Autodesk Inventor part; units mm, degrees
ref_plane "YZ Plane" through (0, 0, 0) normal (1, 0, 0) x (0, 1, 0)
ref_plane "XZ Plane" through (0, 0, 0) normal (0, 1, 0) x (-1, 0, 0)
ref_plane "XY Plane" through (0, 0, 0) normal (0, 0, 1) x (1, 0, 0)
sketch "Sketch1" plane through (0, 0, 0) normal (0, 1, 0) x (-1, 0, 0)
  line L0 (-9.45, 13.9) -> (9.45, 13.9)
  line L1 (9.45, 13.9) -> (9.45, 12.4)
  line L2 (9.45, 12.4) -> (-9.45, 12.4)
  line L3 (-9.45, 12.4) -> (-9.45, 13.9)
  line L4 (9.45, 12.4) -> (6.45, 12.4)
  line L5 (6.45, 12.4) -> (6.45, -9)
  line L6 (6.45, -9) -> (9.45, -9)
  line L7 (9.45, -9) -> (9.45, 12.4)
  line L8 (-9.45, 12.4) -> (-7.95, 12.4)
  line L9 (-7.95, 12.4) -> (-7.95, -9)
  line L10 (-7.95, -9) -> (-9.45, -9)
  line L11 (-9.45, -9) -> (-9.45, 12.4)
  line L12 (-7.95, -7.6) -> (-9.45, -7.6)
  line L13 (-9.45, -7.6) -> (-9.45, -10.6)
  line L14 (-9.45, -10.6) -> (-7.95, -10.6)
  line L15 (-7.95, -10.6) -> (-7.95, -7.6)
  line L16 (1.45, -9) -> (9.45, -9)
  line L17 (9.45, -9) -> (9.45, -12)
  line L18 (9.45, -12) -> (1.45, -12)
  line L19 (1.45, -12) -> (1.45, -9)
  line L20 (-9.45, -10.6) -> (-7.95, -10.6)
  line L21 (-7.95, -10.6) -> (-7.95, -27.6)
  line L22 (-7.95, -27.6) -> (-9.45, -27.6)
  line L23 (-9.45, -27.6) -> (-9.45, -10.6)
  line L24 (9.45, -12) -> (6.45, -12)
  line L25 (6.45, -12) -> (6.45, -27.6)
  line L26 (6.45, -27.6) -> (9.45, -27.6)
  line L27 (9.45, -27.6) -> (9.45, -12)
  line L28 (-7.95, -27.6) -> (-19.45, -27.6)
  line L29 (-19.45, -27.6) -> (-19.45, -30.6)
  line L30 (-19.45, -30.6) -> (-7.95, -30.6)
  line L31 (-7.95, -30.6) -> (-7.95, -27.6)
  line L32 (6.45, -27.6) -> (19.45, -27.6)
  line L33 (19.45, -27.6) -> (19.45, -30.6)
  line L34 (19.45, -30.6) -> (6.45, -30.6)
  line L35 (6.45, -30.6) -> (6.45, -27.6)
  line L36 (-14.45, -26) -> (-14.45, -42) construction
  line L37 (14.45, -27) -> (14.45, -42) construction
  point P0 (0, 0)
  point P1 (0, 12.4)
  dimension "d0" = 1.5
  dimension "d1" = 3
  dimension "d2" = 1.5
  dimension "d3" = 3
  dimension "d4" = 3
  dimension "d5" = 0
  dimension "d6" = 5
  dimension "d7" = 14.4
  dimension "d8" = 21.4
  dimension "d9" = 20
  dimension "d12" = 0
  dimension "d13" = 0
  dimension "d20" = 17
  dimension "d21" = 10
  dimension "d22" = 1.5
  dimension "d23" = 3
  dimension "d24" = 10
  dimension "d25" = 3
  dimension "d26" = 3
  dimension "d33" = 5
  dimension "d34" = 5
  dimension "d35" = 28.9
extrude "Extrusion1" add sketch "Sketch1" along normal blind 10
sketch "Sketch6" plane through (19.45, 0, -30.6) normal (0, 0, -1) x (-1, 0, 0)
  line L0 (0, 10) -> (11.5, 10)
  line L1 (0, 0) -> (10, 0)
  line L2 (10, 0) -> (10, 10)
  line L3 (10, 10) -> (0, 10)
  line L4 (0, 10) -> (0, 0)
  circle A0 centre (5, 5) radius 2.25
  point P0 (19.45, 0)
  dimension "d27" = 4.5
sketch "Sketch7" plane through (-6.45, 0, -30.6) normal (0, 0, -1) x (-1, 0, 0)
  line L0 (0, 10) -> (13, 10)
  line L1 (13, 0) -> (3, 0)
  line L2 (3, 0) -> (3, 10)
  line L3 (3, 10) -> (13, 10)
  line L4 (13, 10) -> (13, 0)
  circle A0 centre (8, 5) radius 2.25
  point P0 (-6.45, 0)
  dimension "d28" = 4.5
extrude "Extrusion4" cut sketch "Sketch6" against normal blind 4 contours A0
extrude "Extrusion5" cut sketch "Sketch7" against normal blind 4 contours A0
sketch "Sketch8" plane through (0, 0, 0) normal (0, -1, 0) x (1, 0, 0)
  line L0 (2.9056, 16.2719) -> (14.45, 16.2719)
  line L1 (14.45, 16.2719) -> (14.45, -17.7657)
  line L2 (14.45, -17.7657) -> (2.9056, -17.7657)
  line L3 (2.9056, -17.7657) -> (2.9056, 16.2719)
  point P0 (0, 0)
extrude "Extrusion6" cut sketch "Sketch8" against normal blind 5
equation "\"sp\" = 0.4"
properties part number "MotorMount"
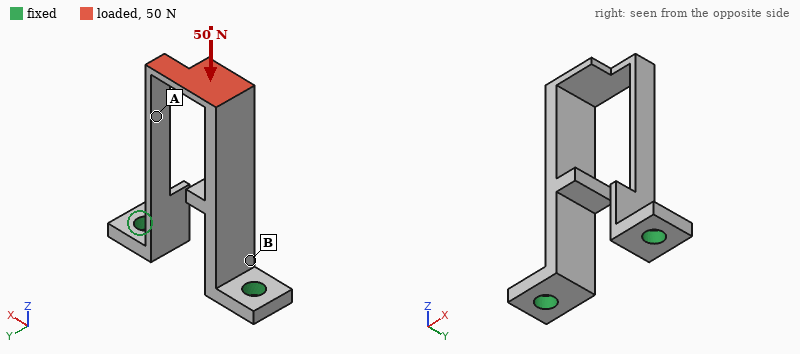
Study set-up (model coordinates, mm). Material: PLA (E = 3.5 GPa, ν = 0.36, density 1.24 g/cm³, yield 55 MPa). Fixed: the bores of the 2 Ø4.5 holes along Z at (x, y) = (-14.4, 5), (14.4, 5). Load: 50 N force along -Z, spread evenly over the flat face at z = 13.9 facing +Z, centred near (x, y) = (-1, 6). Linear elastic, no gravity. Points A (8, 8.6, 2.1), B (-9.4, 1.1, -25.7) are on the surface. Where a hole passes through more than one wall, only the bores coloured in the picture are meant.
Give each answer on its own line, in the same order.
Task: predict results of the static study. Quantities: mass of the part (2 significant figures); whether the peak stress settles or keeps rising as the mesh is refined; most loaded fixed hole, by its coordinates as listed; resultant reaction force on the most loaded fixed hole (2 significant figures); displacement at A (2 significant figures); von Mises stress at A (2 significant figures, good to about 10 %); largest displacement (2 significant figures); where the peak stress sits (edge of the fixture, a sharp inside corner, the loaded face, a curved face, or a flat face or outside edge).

3.2 g
keeps rising
(-14.4, 5)
32 N
0.61 mm
9.2 MPa
0.66 mm
a sharp inside corner
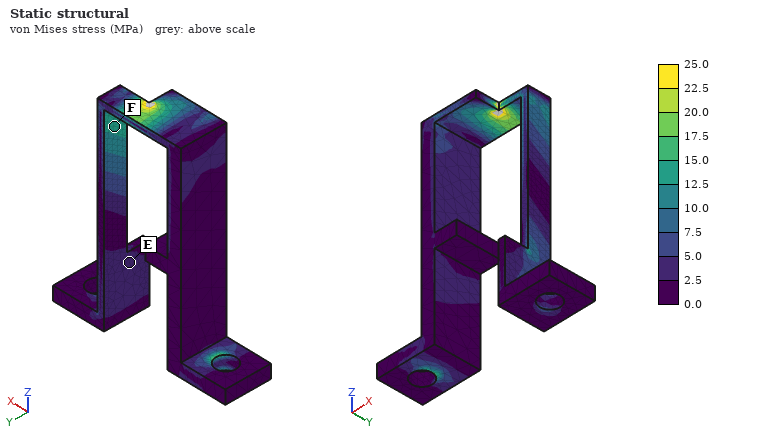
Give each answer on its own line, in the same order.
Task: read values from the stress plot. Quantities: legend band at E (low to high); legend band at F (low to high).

2.5 to 5.0 MPa
12.5 to 15.0 MPa
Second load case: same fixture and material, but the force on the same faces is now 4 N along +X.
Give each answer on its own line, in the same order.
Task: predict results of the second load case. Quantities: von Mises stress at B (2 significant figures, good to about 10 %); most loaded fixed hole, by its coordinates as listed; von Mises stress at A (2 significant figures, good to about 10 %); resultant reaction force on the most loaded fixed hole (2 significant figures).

5.0 MPa
(-14.4, 5)
3.9 MPa
4.9 N
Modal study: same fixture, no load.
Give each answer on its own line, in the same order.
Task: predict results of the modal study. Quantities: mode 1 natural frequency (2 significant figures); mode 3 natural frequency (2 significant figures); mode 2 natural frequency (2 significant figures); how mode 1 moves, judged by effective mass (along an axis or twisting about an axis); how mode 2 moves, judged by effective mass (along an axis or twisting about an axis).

410 Hz
1400 Hz
670 Hz
along X
along Y
